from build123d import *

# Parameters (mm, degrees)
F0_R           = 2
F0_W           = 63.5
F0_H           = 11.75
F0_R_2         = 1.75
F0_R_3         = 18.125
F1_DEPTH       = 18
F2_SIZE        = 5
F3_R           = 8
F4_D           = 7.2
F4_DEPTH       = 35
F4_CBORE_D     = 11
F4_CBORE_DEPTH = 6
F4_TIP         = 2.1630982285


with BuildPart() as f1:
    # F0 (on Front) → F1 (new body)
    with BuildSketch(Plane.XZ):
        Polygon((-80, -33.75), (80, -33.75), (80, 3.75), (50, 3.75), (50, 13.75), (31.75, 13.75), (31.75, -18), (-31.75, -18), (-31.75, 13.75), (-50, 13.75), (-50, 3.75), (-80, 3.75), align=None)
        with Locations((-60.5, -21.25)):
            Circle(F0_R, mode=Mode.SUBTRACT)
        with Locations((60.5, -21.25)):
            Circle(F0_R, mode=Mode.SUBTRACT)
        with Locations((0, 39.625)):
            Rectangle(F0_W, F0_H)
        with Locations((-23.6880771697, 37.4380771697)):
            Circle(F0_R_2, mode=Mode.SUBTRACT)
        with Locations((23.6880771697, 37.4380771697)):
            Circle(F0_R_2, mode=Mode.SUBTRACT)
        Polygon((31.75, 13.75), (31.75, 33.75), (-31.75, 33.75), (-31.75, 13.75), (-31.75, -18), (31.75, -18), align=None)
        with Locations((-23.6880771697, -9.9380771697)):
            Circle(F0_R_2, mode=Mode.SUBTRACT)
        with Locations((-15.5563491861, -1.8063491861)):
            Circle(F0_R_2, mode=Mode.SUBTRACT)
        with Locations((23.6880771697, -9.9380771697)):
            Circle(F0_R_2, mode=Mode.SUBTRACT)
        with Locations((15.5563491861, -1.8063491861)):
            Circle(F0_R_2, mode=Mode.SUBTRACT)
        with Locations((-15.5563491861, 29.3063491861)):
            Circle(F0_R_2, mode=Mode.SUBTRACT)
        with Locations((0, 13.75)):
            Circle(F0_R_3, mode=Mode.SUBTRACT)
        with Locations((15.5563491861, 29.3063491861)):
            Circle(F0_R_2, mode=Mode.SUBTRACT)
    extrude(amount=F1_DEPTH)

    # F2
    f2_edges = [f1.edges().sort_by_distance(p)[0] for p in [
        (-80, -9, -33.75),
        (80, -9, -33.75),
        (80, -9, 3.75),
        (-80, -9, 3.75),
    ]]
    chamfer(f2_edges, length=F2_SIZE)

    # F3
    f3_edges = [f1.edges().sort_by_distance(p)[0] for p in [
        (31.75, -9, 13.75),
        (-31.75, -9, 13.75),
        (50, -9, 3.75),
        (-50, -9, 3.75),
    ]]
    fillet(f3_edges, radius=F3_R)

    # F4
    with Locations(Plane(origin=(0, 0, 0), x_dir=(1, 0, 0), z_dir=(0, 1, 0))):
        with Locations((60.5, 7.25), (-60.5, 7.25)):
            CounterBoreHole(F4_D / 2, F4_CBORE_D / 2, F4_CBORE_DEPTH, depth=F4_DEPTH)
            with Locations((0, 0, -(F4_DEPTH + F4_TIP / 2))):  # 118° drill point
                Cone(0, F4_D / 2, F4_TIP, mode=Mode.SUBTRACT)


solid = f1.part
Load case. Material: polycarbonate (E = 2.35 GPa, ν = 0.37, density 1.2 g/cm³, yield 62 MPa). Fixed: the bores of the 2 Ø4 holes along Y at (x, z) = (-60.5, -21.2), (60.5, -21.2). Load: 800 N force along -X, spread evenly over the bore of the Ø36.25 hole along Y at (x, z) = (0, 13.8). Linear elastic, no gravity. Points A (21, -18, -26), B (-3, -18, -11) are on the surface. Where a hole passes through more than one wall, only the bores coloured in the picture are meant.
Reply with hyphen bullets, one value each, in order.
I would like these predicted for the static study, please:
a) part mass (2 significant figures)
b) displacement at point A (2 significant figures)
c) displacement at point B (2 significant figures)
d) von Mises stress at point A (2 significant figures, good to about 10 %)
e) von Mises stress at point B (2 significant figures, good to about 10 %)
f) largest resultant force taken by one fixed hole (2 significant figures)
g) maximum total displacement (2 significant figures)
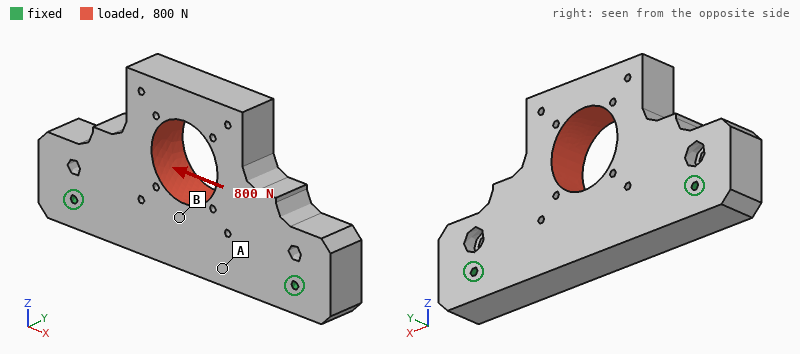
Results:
- 170 g
- 9.9 µm
- 15 µm
- 0.38 MPa
- 0.91 MPa
- 460 N
- 62 µm
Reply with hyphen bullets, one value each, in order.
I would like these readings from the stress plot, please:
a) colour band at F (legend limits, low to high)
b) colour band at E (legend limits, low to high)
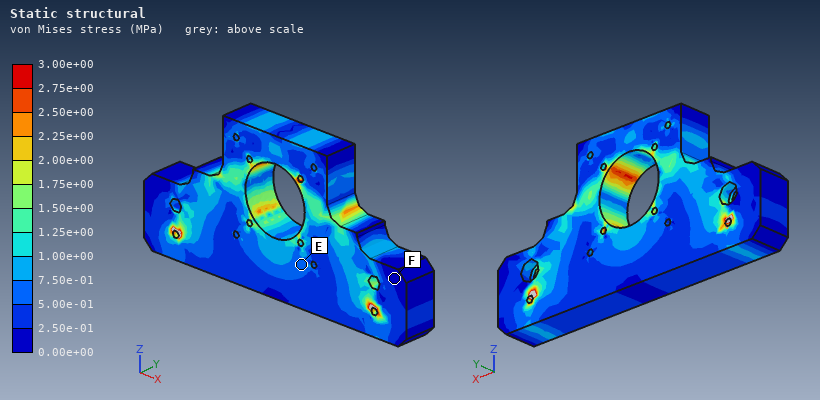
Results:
- 0.00e+00 to 2.50e-01 MPa
- 5.00e-01 to 7.50e-01 MPa
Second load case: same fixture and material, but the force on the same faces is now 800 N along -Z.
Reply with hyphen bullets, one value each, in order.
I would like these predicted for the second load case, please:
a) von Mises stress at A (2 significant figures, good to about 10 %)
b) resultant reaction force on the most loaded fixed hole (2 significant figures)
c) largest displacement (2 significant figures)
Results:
- 0.75 MPa
- 480 N
- 92 µm
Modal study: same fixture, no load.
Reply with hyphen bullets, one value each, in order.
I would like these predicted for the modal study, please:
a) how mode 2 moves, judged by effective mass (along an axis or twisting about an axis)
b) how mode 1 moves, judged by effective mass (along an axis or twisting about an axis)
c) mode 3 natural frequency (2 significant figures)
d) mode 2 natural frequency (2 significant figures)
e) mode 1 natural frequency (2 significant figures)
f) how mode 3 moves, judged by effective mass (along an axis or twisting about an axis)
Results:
- along Y
- along Y
- 1500 Hz
- 1400 Hz
- 590 Hz
- along Z
